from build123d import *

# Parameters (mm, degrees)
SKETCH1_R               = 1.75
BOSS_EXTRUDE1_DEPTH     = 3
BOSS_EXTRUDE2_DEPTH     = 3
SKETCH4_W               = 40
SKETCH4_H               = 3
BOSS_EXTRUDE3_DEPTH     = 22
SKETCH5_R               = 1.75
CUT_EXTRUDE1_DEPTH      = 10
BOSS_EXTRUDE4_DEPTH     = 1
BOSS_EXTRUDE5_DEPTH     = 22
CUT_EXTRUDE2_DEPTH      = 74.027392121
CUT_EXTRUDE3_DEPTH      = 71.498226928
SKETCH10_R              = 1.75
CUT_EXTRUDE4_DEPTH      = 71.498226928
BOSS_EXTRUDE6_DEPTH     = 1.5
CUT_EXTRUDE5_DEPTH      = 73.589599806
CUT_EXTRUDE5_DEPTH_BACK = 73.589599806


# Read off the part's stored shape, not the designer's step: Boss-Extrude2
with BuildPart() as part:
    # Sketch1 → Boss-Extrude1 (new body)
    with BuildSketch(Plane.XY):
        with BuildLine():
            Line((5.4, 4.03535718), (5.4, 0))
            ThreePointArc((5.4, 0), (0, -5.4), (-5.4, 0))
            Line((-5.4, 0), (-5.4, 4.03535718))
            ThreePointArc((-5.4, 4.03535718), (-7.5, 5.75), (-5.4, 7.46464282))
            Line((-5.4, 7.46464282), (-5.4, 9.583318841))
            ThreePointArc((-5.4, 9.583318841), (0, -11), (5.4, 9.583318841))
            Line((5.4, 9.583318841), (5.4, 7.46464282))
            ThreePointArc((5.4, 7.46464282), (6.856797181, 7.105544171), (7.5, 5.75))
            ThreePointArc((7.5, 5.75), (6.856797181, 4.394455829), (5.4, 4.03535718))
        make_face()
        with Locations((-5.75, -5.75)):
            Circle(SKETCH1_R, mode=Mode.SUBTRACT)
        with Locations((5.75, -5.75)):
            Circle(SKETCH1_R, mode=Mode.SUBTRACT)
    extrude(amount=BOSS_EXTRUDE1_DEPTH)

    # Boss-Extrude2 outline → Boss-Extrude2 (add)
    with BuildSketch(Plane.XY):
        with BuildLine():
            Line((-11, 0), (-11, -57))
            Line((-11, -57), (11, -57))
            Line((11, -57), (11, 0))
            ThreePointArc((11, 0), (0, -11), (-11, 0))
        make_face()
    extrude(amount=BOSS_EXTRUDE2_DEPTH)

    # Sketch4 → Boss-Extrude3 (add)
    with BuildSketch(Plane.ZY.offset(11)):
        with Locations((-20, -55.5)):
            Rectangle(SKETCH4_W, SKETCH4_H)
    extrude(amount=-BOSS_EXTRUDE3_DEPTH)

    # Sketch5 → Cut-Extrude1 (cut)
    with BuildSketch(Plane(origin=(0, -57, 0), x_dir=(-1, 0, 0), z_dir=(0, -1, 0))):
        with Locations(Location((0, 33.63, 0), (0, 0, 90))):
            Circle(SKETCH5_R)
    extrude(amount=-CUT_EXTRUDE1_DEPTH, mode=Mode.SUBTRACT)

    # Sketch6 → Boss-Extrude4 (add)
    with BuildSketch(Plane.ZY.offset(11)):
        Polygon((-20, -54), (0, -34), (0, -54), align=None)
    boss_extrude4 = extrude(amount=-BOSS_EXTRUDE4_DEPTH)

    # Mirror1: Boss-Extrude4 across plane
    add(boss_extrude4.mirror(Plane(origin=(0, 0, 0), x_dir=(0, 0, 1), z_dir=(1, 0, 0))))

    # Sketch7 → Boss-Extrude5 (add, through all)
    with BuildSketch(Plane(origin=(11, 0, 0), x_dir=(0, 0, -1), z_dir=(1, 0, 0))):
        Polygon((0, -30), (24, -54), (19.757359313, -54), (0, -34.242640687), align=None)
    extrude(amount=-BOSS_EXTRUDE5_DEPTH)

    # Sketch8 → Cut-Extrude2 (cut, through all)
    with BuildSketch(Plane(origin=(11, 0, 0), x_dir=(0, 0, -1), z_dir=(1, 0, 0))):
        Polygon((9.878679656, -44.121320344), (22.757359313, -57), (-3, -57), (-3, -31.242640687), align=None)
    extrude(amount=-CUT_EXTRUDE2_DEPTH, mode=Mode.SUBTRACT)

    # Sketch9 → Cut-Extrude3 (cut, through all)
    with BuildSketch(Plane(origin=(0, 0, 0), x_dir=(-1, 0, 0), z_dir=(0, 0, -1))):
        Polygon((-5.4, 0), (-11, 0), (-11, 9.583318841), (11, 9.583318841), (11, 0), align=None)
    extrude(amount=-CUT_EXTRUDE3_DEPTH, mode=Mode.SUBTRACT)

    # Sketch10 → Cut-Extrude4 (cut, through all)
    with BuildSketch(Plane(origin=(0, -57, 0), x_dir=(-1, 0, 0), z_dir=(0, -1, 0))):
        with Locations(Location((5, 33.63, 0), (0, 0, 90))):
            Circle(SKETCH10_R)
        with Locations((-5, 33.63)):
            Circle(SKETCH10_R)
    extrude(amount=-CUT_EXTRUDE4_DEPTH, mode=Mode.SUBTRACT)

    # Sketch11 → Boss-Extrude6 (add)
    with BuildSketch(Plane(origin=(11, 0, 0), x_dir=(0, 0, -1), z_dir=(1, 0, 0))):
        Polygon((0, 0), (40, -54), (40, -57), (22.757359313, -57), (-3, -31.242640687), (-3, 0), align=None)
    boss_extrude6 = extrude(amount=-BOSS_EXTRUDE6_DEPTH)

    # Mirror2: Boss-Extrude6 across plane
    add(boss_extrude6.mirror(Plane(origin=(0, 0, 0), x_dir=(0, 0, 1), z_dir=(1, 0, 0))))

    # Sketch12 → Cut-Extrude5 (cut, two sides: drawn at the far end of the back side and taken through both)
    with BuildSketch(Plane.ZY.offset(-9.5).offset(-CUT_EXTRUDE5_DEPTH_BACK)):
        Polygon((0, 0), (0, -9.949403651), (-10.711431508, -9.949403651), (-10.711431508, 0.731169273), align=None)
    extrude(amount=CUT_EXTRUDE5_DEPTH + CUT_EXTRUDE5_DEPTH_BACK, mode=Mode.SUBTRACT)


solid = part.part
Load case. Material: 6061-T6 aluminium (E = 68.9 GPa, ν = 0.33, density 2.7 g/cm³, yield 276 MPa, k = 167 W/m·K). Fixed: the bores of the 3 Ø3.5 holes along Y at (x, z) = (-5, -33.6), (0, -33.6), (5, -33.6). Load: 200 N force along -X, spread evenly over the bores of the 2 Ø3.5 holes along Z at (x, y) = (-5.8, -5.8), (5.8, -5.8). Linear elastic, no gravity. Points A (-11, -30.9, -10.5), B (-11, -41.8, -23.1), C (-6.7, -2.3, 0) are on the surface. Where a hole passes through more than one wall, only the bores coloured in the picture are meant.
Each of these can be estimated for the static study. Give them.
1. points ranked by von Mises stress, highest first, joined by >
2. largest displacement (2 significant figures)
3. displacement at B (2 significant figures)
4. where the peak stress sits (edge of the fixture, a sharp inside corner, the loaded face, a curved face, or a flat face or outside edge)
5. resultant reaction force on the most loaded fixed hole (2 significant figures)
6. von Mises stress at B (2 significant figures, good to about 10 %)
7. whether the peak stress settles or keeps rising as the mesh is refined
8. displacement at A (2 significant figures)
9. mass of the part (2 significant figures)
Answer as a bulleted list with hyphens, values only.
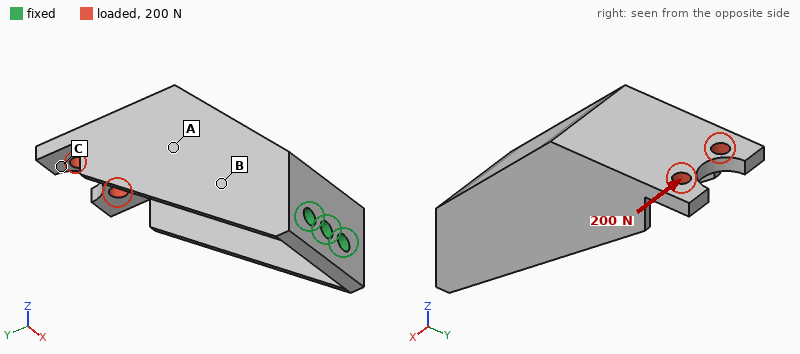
- B > A > C
- 0.78 mm
- 0.15 mm
- edge of the fixture
- 810 N
- 43 MPa
- keeps rising
- 0.32 mm
- 20 g
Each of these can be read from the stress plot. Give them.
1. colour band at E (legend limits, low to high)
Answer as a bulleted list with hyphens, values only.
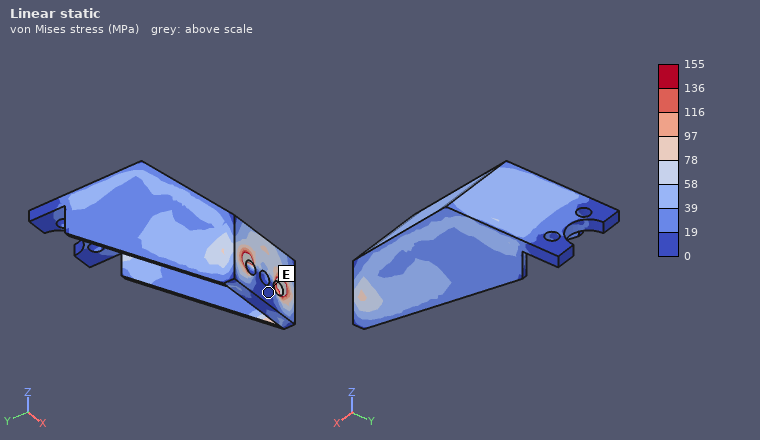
- 0 to 19 MPa
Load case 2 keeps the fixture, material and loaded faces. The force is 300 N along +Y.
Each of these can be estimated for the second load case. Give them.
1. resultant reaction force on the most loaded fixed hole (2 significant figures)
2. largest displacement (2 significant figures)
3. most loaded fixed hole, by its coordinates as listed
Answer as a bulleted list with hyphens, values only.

- 320 N
- 0.43 mm
- (0, -33.6)
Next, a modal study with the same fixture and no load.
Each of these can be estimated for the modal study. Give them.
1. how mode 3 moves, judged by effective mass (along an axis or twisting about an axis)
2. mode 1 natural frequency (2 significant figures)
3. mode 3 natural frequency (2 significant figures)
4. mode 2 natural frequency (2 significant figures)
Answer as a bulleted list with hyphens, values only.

- along X
- 1300 Hz
- 5500 Hz
- 1300 Hz
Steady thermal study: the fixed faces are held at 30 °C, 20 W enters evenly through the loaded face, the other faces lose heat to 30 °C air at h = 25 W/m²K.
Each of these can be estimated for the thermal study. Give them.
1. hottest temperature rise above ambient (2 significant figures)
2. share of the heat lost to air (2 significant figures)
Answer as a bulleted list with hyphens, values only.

- 74 K
- 26 %
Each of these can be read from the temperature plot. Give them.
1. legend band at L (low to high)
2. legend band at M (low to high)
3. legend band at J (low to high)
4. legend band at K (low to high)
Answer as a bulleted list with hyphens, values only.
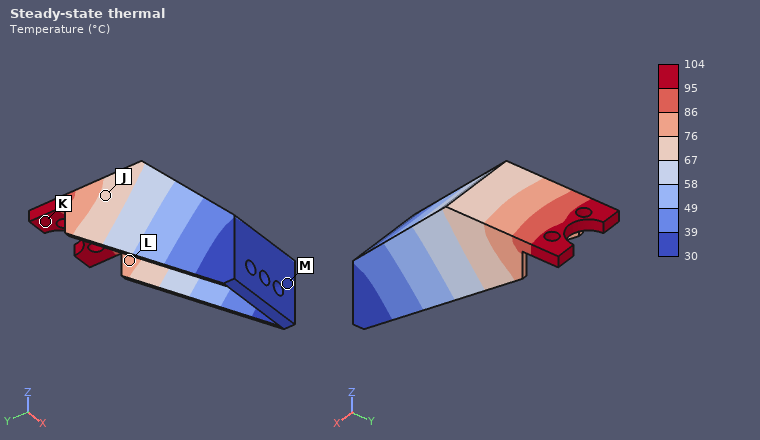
- 76 to 86 °C
- 30 to 39 °C
- 67 to 76 °C
- 95 to 104 °C
